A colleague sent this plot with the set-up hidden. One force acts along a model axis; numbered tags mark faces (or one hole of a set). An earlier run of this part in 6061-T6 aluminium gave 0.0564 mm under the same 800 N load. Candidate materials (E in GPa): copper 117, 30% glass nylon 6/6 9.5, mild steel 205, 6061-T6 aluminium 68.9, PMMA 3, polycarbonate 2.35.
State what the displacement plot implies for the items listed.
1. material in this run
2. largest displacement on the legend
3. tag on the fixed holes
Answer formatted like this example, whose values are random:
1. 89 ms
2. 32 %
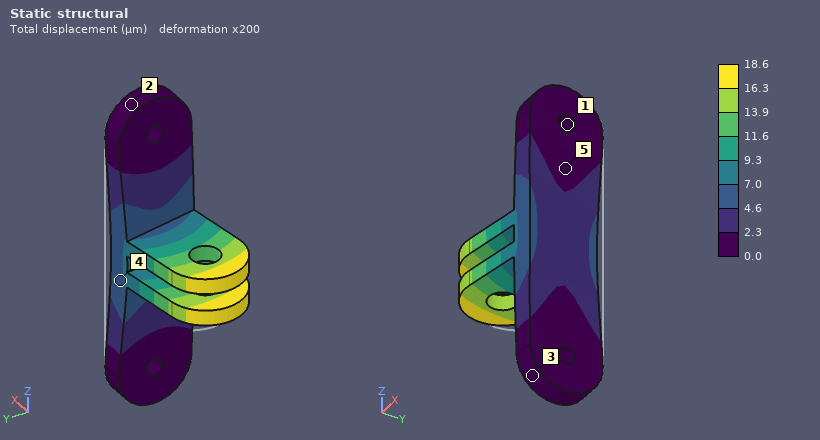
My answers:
1. mild steel
2. 18.6 µm
3. 1
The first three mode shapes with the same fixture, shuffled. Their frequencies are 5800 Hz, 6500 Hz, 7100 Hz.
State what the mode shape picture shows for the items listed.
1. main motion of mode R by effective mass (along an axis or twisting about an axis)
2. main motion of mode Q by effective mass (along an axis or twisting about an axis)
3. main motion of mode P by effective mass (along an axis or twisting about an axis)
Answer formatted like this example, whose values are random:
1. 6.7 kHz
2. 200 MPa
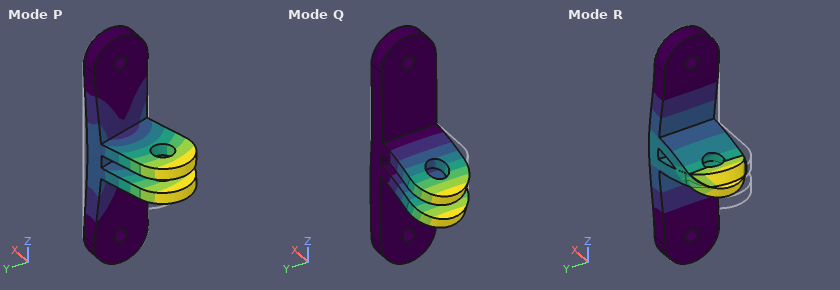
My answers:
1. along X
2. along Z
3. along Y
